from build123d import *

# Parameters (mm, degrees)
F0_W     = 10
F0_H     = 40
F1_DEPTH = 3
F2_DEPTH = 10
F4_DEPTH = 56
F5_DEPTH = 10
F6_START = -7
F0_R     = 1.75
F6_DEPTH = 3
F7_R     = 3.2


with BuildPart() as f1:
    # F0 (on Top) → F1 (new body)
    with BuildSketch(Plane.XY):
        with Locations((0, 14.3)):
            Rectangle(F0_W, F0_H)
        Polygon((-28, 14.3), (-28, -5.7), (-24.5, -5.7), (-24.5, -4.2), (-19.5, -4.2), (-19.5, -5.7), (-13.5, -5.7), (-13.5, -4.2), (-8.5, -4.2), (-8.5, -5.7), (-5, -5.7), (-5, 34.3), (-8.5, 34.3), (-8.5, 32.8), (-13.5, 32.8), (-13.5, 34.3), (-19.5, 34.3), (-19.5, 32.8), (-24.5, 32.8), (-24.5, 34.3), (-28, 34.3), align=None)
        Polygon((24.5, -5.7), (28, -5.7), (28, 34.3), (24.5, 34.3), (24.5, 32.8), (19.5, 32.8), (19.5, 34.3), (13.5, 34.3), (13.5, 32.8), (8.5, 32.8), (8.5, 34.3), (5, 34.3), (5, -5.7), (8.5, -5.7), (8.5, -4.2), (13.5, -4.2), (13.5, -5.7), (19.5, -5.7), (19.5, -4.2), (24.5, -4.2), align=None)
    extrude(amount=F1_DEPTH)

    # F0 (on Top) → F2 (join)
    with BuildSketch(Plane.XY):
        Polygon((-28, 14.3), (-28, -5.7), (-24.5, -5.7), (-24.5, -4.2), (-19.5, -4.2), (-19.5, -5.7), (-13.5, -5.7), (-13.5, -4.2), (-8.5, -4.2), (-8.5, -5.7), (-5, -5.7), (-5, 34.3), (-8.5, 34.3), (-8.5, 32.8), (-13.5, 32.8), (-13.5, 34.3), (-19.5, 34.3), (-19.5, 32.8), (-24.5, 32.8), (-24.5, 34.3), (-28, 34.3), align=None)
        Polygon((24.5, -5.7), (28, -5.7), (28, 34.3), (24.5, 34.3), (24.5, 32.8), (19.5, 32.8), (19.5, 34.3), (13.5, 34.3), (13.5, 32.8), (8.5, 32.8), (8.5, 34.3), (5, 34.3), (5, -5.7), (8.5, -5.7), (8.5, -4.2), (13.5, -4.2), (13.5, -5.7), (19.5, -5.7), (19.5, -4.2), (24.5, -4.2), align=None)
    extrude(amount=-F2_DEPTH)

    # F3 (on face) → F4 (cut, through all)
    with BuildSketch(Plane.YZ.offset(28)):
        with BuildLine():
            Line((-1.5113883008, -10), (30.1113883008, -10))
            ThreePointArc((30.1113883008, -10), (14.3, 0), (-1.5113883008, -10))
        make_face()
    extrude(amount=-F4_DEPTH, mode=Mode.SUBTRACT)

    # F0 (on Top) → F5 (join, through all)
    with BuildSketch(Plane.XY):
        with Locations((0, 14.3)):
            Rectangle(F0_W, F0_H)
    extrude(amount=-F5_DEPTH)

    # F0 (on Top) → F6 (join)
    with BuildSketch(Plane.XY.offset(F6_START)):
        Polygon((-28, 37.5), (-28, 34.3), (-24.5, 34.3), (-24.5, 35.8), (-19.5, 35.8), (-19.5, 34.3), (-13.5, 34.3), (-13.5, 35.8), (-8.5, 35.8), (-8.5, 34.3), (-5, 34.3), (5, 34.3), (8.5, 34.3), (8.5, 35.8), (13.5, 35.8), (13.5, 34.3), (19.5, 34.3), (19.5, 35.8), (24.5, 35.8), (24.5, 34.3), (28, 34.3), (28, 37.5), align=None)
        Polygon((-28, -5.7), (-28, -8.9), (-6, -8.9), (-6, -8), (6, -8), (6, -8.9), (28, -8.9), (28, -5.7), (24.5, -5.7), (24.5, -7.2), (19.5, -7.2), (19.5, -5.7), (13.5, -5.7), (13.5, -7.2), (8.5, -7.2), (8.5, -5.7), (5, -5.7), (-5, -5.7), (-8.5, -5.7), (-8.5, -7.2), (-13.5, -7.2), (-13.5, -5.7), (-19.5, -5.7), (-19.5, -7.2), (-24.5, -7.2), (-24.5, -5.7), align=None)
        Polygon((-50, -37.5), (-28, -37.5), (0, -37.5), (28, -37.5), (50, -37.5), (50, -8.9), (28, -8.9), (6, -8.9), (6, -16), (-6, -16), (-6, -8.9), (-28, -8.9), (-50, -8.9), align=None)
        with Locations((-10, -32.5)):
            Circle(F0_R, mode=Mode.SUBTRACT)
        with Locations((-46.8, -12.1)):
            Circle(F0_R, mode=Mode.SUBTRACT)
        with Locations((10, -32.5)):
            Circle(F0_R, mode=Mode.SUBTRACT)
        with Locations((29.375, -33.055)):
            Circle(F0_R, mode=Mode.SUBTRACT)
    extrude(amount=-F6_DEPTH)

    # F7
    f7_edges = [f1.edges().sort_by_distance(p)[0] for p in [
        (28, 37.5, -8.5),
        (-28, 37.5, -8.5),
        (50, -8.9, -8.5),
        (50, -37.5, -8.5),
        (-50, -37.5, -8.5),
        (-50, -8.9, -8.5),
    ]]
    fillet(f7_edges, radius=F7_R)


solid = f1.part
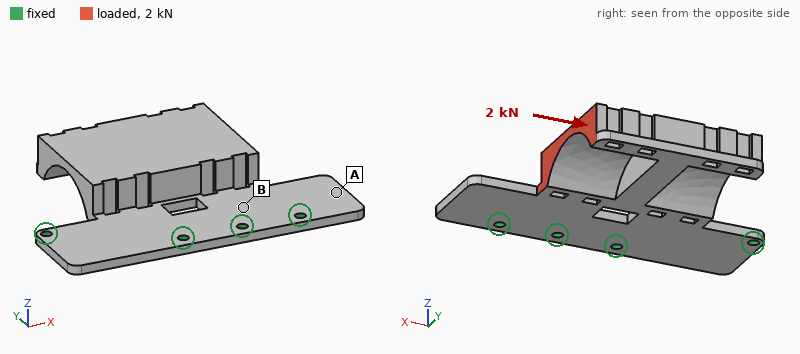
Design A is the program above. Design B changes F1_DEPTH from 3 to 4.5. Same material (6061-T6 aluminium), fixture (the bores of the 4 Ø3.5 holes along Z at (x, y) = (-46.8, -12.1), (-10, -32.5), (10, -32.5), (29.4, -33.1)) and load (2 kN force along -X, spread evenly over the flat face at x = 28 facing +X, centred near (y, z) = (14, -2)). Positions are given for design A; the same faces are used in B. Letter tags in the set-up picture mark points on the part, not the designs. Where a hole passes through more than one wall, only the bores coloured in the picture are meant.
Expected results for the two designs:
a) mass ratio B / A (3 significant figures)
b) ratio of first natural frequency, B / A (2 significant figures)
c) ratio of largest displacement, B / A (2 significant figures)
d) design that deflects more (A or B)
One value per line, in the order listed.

1.12
0.92
1.2
B
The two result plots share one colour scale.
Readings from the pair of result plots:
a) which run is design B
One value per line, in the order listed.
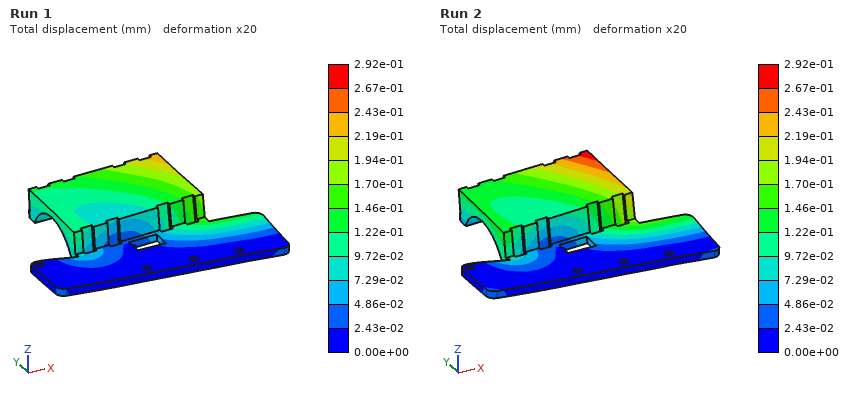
Run 2
